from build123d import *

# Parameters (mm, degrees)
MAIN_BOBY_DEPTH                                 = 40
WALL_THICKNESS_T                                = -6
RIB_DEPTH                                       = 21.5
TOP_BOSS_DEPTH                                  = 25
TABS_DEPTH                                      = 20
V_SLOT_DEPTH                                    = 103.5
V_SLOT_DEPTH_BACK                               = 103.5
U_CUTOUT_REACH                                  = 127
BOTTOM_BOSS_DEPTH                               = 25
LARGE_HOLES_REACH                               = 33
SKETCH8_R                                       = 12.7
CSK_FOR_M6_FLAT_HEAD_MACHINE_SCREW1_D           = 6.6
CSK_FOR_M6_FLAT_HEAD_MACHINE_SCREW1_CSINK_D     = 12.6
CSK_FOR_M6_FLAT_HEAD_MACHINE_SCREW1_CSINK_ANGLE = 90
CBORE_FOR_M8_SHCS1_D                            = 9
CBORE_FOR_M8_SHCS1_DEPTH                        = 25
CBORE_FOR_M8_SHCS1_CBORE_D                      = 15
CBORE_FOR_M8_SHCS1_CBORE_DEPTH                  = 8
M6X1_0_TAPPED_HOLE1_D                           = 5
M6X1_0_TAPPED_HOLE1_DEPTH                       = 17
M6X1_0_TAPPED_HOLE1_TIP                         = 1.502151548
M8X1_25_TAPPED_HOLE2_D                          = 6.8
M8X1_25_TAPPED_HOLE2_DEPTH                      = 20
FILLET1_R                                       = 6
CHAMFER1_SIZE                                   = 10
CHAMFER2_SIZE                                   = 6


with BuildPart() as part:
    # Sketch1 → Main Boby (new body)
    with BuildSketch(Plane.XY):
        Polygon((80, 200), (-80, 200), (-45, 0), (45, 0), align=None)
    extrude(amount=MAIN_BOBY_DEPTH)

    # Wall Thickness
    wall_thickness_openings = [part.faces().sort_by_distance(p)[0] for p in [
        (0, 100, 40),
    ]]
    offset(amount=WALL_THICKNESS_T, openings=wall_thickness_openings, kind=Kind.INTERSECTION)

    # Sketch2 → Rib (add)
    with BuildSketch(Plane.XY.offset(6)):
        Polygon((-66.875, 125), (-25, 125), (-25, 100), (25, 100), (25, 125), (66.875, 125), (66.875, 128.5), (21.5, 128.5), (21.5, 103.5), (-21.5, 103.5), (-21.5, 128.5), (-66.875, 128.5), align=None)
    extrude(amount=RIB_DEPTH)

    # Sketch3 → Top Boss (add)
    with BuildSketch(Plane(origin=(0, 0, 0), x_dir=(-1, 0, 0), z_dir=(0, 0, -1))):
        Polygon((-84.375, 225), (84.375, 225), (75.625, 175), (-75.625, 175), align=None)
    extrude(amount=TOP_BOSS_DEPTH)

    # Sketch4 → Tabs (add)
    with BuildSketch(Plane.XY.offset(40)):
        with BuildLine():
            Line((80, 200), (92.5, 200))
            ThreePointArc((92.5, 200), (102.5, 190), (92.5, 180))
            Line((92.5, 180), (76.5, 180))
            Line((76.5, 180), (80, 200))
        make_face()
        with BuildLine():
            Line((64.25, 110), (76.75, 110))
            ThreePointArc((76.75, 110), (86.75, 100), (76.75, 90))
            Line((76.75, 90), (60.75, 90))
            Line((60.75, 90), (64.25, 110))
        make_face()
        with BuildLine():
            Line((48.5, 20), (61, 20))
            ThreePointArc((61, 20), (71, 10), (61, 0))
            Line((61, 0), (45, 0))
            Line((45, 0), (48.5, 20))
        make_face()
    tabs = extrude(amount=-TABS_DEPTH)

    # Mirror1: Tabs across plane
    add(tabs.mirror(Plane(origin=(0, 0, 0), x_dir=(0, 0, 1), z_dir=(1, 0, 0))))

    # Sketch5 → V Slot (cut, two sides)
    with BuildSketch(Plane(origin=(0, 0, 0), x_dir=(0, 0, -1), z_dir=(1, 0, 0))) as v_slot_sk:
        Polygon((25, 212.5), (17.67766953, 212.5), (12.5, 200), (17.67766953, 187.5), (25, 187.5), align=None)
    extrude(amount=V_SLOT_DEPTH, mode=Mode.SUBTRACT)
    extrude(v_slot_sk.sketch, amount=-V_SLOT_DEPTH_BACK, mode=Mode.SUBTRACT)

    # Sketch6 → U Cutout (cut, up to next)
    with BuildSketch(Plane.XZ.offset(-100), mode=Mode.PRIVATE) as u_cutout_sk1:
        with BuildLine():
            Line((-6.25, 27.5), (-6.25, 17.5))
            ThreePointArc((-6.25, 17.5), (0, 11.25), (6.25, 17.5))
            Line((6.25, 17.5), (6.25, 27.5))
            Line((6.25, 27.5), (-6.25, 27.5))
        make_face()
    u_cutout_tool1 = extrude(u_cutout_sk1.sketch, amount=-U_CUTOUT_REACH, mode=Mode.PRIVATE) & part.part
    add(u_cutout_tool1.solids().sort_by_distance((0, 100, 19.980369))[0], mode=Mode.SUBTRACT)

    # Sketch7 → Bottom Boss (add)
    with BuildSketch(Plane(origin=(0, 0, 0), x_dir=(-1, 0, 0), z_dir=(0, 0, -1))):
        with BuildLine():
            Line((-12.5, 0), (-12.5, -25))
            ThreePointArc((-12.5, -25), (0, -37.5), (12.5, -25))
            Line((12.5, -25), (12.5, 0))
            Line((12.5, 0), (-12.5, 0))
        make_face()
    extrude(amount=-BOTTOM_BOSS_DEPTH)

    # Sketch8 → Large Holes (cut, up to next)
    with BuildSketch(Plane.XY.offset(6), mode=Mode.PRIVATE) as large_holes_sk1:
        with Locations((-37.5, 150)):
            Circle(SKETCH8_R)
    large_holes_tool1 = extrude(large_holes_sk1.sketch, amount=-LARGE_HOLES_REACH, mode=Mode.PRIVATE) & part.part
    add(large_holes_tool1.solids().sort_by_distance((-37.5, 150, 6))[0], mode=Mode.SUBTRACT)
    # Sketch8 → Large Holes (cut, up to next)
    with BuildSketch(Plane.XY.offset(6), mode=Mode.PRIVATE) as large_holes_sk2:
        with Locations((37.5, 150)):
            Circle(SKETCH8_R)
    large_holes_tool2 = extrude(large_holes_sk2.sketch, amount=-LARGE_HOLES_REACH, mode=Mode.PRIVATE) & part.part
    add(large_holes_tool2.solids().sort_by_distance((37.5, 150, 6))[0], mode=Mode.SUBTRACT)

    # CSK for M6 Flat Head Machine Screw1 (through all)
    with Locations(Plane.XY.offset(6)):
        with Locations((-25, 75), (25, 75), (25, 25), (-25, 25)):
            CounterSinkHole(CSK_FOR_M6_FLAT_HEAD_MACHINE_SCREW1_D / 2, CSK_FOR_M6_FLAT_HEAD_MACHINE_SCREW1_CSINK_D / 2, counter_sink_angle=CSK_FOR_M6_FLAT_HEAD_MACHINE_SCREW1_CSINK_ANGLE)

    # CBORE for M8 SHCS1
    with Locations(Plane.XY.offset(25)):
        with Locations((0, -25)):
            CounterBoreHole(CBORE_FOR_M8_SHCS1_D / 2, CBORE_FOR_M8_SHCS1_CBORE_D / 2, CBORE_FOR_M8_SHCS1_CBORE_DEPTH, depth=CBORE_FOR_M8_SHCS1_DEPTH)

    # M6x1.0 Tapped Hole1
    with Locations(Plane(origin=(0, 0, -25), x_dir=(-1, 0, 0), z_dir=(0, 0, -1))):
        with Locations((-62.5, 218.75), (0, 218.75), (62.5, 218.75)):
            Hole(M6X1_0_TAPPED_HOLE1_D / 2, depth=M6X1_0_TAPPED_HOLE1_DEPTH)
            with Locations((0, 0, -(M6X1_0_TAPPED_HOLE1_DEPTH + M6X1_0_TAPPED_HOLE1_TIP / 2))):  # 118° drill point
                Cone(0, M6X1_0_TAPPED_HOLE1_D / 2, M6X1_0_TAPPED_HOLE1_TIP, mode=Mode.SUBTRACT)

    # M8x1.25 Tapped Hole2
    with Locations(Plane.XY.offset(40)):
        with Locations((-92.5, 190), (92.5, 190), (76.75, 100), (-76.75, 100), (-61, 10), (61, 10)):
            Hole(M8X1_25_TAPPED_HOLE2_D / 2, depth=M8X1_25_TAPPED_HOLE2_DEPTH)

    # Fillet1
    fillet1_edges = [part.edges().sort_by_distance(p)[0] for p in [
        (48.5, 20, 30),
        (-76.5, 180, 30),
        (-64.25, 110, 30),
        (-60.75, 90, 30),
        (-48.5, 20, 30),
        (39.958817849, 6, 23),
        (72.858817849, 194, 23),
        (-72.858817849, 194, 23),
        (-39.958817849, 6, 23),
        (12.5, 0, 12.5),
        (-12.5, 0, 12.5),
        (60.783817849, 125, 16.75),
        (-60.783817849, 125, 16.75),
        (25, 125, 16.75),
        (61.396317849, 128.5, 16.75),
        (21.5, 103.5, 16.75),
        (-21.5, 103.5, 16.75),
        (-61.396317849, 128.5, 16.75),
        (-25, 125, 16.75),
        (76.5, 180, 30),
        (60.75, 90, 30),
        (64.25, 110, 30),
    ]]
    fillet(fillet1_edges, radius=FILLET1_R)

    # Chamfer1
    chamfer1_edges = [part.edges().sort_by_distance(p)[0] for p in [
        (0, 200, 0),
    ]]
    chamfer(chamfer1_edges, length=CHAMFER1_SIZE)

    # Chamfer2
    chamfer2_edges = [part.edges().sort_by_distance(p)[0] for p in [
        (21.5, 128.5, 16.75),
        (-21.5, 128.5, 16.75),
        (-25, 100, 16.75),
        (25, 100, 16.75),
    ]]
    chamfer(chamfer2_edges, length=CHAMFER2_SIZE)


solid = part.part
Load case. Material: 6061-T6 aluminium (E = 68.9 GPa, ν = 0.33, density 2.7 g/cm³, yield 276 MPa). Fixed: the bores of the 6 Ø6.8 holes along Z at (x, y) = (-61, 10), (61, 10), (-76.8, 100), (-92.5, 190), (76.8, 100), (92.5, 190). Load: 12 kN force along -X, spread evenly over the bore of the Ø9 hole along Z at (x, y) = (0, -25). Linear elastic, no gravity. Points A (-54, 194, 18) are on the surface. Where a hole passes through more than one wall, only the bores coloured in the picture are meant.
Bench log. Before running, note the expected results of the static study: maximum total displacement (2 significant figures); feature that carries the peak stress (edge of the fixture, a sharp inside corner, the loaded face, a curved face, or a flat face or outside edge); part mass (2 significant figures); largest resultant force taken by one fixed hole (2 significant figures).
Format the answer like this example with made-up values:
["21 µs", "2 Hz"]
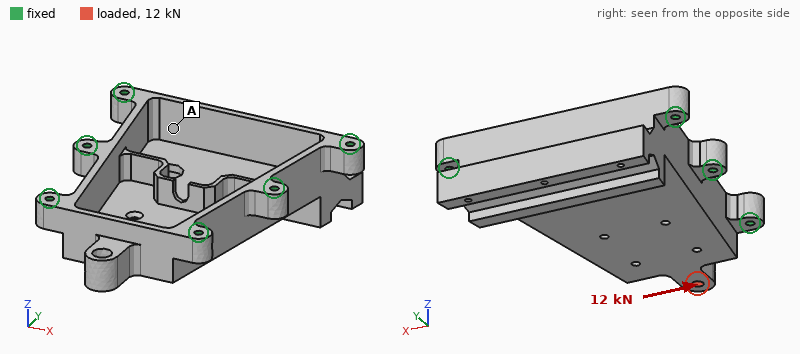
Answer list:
["0.24 mm", "a curved face", "1.4 kg", "6.4 kN"]
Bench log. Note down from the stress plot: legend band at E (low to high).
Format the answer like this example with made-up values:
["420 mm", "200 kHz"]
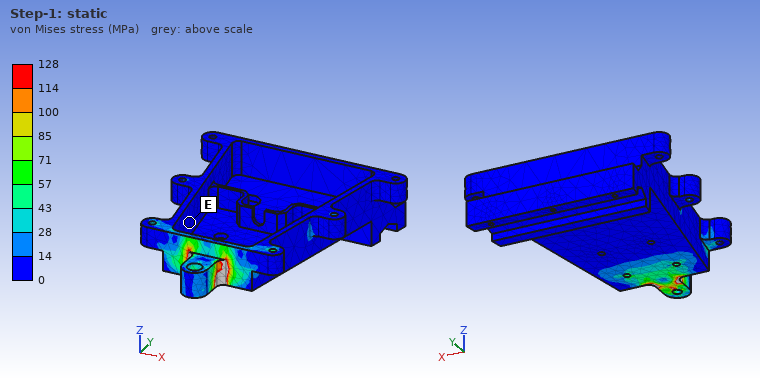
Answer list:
["0 to 14 MPa"]
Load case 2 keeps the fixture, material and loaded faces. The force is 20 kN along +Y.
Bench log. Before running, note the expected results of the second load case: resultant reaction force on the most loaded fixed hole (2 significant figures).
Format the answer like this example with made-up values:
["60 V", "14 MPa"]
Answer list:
["4.8 kN"]
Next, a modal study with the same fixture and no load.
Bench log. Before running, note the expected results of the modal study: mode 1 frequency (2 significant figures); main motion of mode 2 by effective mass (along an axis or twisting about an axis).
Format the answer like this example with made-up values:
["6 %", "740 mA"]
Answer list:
["2500 Hz", "along Z"]
